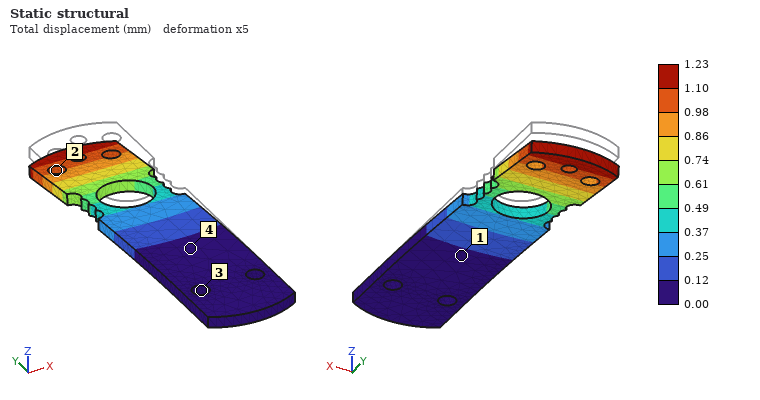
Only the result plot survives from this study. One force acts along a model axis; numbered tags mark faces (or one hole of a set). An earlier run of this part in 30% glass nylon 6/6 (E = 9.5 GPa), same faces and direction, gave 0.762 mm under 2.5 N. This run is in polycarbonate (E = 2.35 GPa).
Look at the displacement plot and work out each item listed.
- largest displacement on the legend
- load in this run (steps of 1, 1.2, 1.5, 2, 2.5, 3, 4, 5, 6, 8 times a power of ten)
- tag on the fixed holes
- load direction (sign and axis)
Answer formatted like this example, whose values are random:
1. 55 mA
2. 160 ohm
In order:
1. 1.23 mm
2. 1 N
3. 3
4. -Z
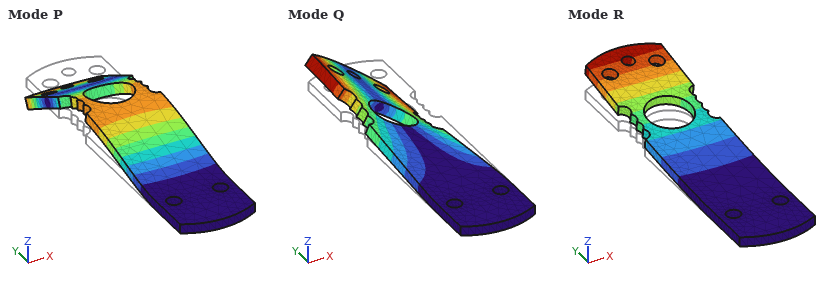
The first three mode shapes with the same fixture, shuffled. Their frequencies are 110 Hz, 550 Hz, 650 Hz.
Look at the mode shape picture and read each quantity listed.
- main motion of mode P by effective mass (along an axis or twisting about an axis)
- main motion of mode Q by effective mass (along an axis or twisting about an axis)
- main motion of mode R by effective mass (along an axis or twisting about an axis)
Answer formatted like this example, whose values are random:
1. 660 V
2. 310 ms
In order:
1. along Z
2. twisting about Y
3. along Z
